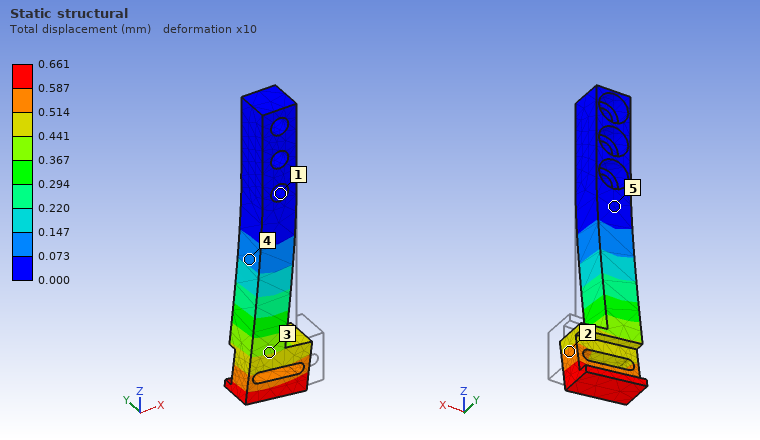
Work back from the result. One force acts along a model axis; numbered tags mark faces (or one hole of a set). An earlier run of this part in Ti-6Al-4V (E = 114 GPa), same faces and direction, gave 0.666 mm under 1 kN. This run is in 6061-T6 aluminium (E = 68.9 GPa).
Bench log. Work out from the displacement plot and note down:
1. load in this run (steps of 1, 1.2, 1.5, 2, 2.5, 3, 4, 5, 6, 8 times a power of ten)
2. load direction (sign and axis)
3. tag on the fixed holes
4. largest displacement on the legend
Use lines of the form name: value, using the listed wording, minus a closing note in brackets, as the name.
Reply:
load in this run: 600 N
load direction: -X
tag on the fixed holes: 1
largest displacement on the legend: 0.661 mm
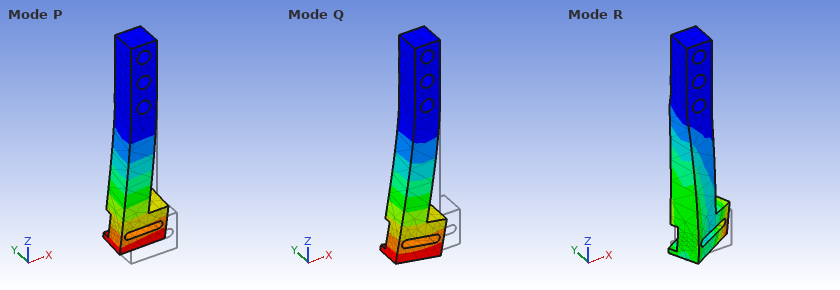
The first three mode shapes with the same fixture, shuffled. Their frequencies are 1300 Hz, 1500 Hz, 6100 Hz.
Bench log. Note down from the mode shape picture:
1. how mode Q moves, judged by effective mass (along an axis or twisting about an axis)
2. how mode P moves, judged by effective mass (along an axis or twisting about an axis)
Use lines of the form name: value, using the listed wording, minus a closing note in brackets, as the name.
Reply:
how mode Q moves, judged by effective mass: along X
how mode P moves, judged by effective mass: along Y
